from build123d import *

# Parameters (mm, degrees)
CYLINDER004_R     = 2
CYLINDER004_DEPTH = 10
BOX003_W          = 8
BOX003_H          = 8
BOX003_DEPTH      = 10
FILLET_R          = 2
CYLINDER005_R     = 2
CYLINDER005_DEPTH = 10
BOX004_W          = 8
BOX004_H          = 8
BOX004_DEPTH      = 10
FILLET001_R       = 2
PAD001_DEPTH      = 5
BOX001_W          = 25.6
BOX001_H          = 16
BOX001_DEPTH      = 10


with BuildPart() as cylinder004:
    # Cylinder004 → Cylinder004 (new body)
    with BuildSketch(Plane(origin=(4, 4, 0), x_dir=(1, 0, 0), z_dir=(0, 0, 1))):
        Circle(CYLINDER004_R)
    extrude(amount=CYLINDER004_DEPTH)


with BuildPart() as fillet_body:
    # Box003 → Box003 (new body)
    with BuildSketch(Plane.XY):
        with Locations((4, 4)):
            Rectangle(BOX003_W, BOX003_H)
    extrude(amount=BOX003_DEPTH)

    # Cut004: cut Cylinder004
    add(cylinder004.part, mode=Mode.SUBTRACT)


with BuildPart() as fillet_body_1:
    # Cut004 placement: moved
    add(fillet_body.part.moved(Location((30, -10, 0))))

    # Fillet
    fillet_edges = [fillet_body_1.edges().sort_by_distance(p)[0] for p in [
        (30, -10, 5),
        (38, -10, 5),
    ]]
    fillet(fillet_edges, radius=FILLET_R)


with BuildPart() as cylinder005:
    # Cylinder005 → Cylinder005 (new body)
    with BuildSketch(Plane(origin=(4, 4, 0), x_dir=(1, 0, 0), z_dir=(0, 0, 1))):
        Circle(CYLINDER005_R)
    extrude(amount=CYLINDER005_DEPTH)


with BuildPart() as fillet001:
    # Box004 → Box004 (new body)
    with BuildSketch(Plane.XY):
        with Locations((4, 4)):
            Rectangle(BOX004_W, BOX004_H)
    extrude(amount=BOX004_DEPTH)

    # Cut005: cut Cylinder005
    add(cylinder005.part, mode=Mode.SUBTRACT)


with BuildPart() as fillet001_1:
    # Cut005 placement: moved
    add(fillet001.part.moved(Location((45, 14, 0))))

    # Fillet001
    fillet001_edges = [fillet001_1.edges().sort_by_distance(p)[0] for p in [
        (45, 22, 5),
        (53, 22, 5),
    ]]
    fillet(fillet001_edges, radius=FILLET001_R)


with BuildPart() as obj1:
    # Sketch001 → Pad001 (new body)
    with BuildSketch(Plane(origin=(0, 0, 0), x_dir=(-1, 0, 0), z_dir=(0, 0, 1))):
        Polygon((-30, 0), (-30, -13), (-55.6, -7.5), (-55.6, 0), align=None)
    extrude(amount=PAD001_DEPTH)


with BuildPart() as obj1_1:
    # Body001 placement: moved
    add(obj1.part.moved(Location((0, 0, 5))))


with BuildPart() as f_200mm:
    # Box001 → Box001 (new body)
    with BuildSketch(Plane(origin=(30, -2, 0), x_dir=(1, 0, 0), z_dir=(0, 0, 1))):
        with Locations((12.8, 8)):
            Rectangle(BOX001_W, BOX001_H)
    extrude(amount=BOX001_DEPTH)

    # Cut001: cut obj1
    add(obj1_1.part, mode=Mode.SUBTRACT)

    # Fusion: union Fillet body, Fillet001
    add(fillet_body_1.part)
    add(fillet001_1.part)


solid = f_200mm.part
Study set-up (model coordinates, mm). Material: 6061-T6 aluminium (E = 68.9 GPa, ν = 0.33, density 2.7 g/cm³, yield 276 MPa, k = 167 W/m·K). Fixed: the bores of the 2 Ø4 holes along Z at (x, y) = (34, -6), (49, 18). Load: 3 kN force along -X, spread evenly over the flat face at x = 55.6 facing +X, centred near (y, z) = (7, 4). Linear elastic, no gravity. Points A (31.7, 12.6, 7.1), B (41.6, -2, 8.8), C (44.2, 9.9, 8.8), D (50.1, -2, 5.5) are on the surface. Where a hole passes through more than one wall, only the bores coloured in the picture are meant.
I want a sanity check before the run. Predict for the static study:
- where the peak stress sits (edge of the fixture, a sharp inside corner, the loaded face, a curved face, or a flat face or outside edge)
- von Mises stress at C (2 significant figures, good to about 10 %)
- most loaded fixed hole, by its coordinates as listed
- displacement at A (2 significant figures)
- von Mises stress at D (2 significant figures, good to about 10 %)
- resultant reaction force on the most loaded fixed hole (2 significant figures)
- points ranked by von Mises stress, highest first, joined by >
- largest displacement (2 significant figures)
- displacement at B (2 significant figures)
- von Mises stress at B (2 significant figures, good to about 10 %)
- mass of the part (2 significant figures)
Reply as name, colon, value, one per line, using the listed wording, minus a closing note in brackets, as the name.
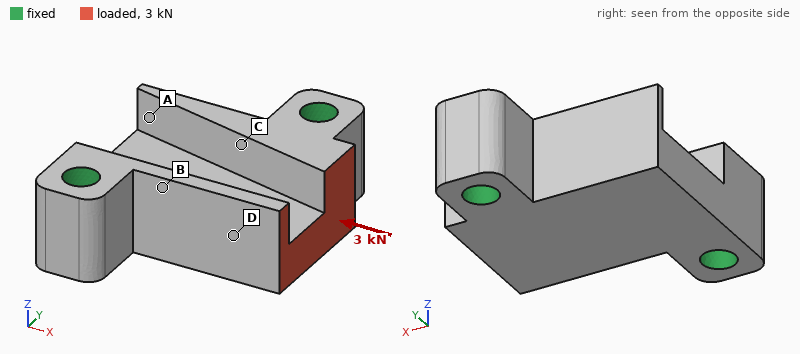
where the peak stress sits: edge of the fixture
von Mises stress at C: 23 MPa
most loaded fixed hole, by its coordinates as listed: (49, 18)
displacement at A: 7.1 µm
von Mises stress at D: 30 MPa
resultant reaction force on the most loaded fixed hole: 1.7 kN
points ranked by von Mises stress, highest first, joined by >: B > D > C > A
largest displacement: 18 µm
displacement at B: 6.7 µm
von Mises stress at B: 45 MPa
mass of the part: 10 g
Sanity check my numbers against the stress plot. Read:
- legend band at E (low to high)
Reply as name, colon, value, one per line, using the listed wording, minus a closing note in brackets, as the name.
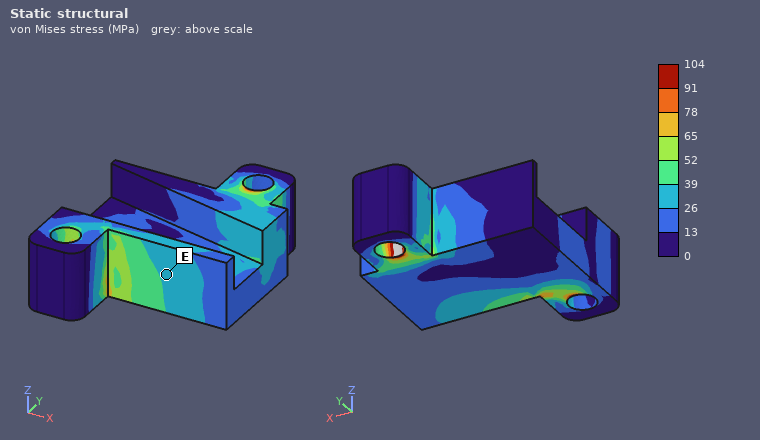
legend band at E: 26 to 39 MPa
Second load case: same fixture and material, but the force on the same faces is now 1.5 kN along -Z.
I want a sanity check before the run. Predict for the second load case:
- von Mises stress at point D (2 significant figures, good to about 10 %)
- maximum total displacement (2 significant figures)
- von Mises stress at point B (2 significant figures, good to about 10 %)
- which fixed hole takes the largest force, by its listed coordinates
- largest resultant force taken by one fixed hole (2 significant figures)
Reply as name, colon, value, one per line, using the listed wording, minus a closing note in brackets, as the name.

von Mises stress at point D: 35 MPa
maximum total displacement: 61 µm
von Mises stress at point B: 59 MPa
which fixed hole takes the largest force, by its listed coordinates: (49, 18)
largest resultant force taken by one fixed hole: 1.4 kN
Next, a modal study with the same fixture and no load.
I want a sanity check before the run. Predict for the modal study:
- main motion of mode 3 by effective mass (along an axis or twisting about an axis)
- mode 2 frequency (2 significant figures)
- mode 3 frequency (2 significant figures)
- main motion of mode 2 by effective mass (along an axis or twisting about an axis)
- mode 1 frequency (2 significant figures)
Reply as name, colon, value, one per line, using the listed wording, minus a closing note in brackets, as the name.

main motion of mode 3 by effective mass: along X
mode 2 frequency: 24 kHz
mode 3 frequency: 34 kHz
main motion of mode 2 by effective mass: along Z
mode 1 frequency: 20 kHz
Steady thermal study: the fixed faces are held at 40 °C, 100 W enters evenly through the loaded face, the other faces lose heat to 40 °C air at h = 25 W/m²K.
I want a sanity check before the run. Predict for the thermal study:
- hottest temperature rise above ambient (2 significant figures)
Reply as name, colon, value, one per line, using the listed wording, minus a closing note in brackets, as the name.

hottest temperature rise above ambient: 78 K
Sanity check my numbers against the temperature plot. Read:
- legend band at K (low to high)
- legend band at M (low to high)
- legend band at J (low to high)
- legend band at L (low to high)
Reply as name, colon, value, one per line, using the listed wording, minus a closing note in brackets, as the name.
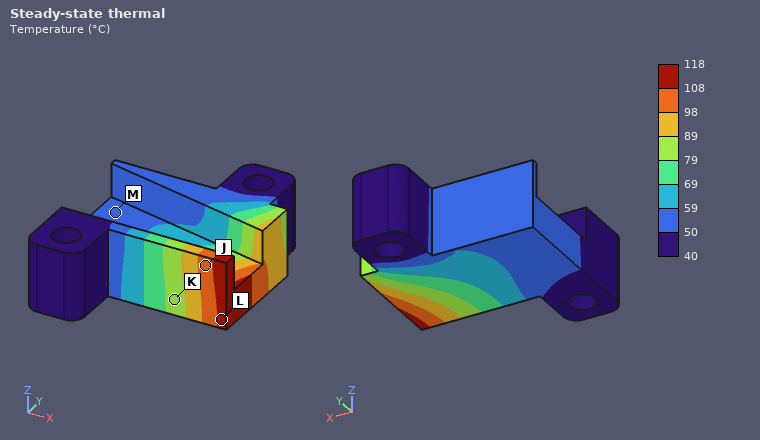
legend band at K: 79 to 89 °C
legend band at M: 50 to 59 °C
legend band at J: 98 to 108 °C
legend band at L: 108 to 118 °C
